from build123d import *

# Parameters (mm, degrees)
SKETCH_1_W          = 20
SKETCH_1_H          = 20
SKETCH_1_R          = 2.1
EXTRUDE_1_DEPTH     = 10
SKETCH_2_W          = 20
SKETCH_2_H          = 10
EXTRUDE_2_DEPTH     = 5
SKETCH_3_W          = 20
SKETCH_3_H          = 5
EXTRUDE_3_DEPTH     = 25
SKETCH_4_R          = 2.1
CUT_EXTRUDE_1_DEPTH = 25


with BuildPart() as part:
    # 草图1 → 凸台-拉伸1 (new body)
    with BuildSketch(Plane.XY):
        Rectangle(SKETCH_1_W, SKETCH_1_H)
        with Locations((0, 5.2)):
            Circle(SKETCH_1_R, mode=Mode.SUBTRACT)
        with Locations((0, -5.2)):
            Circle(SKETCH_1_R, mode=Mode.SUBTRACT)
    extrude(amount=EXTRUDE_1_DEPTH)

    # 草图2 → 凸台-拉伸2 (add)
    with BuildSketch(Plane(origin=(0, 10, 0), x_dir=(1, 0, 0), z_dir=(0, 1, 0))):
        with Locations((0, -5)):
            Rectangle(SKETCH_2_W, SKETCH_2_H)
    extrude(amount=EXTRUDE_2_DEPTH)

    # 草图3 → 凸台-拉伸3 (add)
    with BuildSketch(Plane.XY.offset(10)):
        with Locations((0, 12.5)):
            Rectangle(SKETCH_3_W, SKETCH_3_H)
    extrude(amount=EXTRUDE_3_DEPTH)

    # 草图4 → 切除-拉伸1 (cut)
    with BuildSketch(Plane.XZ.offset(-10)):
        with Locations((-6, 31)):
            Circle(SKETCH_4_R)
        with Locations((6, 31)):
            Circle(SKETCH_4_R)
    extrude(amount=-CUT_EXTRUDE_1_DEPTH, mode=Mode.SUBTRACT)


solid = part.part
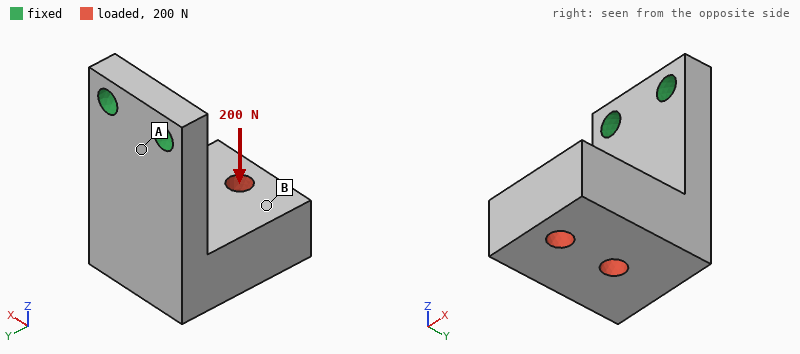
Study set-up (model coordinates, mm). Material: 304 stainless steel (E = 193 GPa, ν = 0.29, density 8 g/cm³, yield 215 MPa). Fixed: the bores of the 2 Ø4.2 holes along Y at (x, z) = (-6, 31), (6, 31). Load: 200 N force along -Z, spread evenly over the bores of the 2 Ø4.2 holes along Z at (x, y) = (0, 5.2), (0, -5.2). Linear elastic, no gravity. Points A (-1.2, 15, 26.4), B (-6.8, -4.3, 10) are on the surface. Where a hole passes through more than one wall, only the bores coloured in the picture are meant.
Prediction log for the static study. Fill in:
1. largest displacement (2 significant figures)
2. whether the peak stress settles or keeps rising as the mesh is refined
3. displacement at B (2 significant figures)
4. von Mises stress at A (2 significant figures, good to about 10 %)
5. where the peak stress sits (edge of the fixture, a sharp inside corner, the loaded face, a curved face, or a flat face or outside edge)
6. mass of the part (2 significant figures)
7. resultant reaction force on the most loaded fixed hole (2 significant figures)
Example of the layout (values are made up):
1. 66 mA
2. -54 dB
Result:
1. 41 µm
2. keeps rising
3. 26 µm
4. 23 MPa
5. edge of the fixture
6. 57 g
7. 100 N
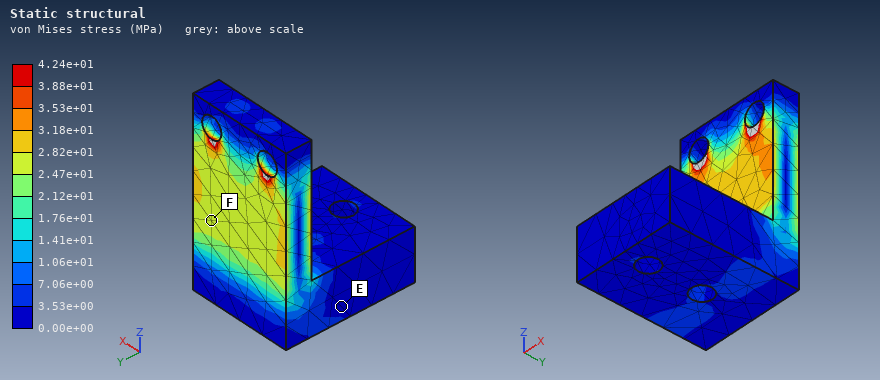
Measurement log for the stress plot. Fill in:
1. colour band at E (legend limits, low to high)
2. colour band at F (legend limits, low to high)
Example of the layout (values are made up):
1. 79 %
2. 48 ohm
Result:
1. 0.00e+00 to 3.53e+00 MPa
2. 2.47e+01 to 2.82e+01 MPa
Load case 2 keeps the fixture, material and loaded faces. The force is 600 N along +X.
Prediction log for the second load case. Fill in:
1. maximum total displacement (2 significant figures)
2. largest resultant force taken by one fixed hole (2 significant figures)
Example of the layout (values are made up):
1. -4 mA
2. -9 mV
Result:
1. 59 µm
2. 1.2 kN
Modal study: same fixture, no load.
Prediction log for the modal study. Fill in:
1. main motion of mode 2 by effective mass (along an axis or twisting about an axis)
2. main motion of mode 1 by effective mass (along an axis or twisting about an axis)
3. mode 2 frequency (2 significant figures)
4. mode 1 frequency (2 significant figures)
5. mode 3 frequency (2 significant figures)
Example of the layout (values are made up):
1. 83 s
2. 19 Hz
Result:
1. along X
2. along Y
3. 3300 Hz
4. 1800 Hz
5. 7000 Hz
